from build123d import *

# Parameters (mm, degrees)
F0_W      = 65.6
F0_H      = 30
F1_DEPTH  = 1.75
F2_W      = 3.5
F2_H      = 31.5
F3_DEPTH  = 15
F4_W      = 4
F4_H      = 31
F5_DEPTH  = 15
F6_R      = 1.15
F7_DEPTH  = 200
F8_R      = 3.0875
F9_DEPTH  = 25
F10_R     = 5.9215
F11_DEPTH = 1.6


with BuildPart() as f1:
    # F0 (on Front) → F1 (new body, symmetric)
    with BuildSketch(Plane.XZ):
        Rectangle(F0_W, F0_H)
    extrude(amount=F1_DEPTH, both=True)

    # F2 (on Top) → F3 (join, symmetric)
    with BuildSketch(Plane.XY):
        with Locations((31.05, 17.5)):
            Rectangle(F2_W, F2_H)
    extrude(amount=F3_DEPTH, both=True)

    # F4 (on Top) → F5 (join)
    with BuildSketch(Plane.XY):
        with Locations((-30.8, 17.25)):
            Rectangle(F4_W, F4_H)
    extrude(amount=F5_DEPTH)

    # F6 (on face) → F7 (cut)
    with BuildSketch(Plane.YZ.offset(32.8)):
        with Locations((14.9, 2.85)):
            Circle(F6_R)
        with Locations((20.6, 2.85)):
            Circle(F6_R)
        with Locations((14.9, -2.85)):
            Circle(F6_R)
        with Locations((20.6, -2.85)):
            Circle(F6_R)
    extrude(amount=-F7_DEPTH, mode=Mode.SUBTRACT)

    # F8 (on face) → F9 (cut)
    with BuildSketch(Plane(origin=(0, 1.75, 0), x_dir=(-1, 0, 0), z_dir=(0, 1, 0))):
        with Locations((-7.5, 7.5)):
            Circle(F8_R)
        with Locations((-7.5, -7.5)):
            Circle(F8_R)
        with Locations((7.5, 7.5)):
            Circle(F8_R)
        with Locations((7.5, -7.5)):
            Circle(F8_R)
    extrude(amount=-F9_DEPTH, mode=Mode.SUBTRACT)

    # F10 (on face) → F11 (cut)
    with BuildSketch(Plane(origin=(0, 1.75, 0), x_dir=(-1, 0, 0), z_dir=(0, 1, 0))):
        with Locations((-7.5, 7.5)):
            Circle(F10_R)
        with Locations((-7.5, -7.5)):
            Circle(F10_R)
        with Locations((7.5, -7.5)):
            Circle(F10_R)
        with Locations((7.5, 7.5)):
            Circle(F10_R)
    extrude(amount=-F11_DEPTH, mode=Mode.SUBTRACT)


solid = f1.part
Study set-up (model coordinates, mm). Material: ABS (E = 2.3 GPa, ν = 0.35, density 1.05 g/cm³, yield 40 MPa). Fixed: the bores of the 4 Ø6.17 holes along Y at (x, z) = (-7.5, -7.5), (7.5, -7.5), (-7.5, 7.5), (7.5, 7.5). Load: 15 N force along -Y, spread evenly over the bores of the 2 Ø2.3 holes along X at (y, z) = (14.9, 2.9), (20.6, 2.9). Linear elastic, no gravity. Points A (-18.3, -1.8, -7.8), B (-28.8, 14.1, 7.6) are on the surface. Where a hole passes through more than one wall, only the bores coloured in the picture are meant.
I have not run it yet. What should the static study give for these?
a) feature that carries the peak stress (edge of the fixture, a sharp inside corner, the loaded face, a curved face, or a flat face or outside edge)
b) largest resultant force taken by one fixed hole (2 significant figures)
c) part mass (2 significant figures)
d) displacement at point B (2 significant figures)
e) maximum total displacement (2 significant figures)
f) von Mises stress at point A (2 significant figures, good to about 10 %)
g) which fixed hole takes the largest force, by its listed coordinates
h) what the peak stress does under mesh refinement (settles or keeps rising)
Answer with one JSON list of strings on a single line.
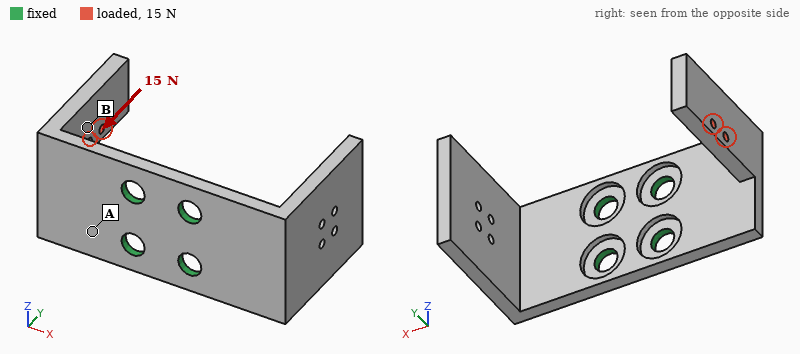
["edge of the fixture", "16 N", "12 g", "0.46 mm", "0.85 mm", "3.0 MPa", "(-7.5, 7.5)", "keeps rising"]
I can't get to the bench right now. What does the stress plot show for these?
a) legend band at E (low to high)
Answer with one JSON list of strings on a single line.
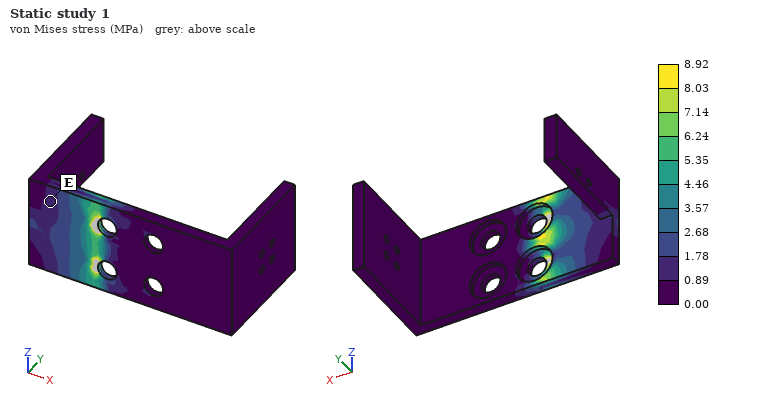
["0.89 to 1.78 MPa"]
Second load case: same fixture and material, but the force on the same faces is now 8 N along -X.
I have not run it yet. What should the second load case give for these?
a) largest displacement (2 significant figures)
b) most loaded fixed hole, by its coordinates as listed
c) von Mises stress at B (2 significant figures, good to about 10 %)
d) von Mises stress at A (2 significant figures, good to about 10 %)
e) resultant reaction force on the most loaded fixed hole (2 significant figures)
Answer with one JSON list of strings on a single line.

["0.80 mm", "(7.5, 7.5)", "1.1 MPa", "2.0 MPa", "5.3 N"]
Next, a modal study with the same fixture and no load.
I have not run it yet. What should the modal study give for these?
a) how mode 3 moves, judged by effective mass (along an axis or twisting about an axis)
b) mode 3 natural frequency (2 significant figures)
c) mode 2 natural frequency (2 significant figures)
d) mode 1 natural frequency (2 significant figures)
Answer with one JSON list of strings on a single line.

["along Z", "580 Hz", "390 Hz", "310 Hz"]
